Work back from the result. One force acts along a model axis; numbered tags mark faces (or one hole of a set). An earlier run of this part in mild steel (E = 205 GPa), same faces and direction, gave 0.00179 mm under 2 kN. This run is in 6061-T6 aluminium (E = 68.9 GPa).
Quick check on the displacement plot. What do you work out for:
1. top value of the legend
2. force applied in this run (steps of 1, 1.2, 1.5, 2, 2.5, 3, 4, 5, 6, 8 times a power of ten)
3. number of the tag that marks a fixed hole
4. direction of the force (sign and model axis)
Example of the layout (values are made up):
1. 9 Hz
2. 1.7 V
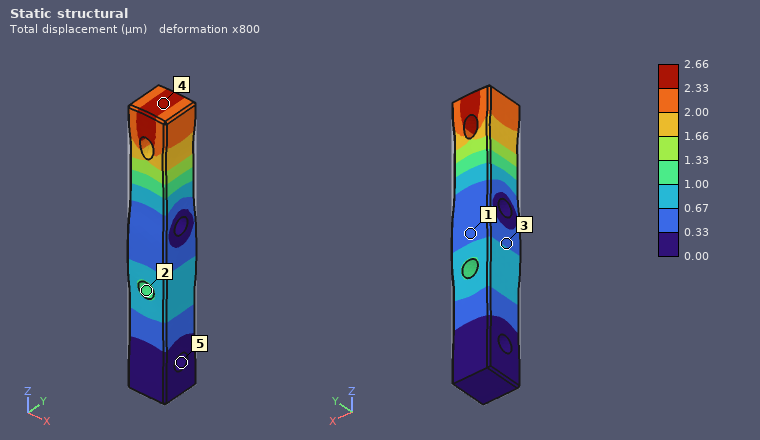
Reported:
1. 2.66 µm
2. 1 kN
3. 5
4. +Z
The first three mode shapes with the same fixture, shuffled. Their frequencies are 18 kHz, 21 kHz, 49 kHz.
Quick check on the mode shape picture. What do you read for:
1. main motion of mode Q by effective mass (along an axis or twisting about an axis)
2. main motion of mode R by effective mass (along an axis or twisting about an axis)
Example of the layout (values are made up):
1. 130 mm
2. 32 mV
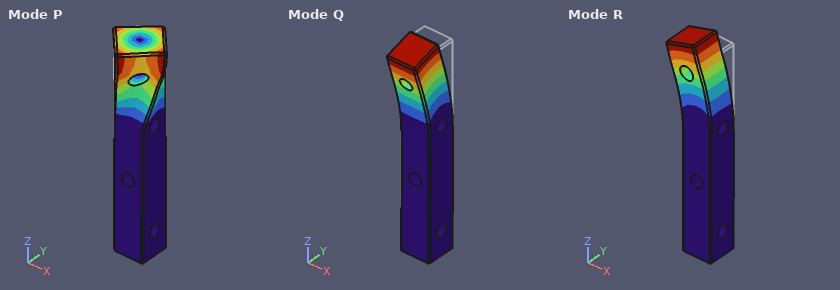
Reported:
1. along Y
2. along X
